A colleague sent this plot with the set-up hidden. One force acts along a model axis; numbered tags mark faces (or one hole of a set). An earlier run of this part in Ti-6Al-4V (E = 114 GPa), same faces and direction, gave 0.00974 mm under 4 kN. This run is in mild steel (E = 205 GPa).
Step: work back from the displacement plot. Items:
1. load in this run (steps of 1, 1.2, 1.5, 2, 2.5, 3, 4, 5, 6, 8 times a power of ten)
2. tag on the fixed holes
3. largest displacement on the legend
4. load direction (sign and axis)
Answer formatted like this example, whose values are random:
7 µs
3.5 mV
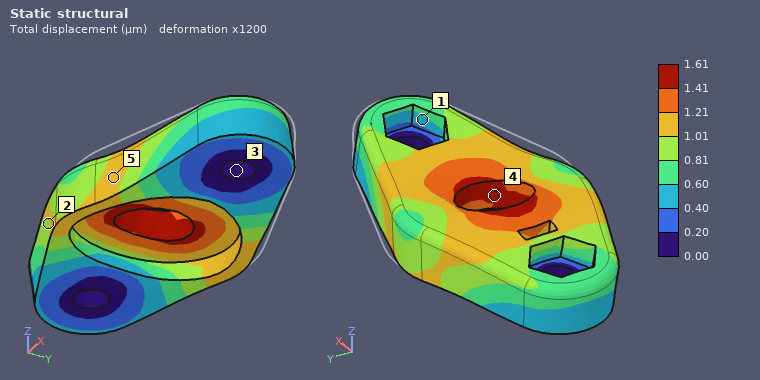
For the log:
1.2 kN
3
1.61 µm
-X
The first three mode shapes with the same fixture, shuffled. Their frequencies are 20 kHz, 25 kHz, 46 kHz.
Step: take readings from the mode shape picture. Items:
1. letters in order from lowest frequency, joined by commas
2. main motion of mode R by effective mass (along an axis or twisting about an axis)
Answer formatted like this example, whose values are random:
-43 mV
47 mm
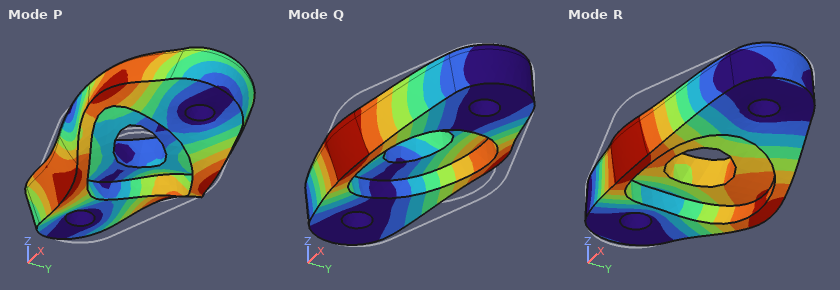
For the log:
Q, R, P
along Z
